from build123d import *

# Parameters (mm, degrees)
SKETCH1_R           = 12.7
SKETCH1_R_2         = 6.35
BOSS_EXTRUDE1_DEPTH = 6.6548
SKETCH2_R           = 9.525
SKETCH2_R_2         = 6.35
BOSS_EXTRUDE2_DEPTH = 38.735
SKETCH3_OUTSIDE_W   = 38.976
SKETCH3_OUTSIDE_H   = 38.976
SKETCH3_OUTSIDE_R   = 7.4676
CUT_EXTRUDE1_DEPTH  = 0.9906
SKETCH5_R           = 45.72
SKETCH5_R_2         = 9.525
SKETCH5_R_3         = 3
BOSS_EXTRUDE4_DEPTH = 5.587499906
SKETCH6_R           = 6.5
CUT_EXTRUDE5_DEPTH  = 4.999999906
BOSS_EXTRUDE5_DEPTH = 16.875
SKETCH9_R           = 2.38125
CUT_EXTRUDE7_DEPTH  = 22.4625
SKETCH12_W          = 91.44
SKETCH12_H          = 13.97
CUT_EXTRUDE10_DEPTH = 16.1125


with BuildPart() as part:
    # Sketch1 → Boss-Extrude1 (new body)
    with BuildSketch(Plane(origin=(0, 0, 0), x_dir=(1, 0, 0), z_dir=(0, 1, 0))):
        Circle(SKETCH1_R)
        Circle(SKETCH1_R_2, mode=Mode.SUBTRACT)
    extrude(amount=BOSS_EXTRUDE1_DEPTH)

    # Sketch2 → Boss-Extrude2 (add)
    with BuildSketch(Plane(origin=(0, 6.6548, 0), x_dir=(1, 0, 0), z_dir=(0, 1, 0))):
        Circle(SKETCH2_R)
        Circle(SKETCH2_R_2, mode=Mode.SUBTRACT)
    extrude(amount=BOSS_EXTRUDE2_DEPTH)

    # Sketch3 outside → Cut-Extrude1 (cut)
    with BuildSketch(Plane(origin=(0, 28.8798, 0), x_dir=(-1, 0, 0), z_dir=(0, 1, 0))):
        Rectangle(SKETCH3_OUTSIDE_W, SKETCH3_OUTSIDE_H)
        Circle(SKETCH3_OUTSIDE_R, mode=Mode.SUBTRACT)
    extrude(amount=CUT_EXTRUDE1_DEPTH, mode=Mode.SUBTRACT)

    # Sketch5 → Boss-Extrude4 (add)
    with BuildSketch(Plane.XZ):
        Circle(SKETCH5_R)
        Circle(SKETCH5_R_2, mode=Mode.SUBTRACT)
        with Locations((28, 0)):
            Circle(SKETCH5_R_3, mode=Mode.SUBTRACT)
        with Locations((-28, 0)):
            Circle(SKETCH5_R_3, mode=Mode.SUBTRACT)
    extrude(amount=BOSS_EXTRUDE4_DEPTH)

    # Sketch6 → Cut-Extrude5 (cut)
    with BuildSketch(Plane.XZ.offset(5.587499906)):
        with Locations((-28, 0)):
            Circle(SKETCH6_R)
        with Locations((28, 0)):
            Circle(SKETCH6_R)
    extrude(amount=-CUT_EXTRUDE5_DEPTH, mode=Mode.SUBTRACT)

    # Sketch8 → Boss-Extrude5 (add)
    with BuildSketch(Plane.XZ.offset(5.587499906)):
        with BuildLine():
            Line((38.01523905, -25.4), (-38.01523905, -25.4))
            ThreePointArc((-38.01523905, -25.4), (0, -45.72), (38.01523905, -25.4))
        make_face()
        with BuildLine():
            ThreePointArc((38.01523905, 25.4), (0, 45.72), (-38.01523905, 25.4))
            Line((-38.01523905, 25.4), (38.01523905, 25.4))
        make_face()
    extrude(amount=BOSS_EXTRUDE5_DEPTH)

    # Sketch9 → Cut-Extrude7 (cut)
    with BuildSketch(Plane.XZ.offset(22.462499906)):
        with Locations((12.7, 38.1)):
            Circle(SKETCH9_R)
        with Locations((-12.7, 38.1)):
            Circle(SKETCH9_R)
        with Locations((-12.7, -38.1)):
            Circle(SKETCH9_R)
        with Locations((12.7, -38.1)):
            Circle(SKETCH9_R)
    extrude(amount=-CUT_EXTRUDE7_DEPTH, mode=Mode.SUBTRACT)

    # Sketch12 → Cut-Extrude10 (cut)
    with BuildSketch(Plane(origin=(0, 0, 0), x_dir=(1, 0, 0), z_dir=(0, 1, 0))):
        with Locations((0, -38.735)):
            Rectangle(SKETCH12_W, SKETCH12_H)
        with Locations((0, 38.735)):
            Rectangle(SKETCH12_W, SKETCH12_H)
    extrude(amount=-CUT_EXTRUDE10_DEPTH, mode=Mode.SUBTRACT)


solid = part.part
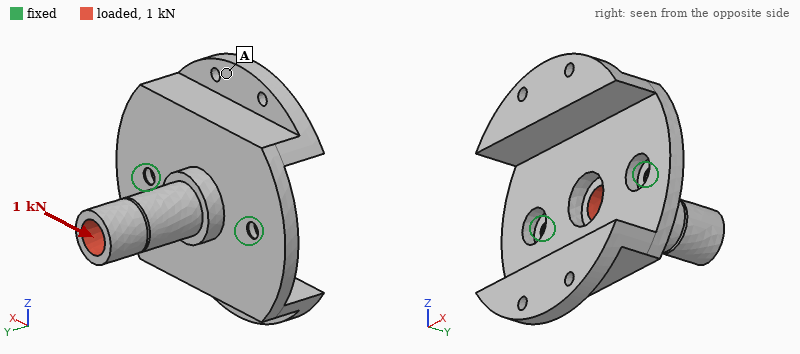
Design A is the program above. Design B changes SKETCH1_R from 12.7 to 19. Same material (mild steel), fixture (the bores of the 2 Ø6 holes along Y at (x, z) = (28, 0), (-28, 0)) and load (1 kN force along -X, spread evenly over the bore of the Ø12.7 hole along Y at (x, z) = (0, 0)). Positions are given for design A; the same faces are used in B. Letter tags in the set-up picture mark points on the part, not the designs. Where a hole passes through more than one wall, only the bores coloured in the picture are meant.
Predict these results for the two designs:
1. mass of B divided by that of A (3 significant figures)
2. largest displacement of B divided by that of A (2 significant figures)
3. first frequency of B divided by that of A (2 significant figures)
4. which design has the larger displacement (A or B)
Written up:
1.07
0.75
1.0
A
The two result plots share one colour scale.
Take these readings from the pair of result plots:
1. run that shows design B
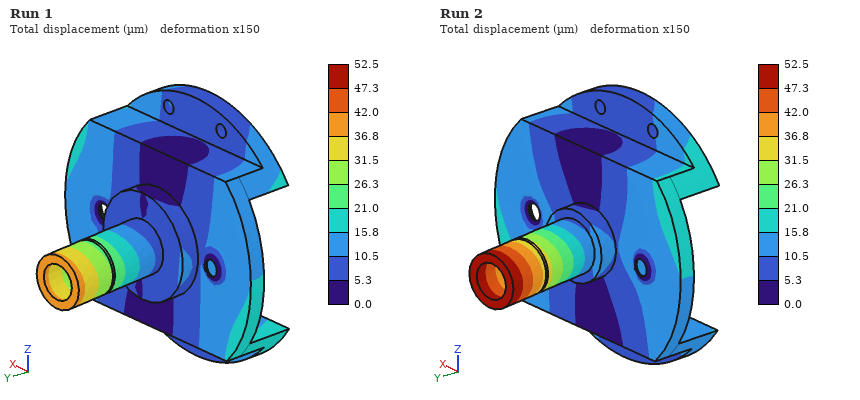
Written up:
Run 1
